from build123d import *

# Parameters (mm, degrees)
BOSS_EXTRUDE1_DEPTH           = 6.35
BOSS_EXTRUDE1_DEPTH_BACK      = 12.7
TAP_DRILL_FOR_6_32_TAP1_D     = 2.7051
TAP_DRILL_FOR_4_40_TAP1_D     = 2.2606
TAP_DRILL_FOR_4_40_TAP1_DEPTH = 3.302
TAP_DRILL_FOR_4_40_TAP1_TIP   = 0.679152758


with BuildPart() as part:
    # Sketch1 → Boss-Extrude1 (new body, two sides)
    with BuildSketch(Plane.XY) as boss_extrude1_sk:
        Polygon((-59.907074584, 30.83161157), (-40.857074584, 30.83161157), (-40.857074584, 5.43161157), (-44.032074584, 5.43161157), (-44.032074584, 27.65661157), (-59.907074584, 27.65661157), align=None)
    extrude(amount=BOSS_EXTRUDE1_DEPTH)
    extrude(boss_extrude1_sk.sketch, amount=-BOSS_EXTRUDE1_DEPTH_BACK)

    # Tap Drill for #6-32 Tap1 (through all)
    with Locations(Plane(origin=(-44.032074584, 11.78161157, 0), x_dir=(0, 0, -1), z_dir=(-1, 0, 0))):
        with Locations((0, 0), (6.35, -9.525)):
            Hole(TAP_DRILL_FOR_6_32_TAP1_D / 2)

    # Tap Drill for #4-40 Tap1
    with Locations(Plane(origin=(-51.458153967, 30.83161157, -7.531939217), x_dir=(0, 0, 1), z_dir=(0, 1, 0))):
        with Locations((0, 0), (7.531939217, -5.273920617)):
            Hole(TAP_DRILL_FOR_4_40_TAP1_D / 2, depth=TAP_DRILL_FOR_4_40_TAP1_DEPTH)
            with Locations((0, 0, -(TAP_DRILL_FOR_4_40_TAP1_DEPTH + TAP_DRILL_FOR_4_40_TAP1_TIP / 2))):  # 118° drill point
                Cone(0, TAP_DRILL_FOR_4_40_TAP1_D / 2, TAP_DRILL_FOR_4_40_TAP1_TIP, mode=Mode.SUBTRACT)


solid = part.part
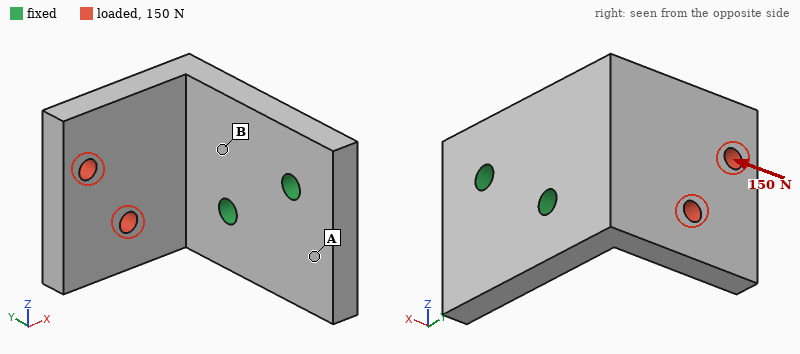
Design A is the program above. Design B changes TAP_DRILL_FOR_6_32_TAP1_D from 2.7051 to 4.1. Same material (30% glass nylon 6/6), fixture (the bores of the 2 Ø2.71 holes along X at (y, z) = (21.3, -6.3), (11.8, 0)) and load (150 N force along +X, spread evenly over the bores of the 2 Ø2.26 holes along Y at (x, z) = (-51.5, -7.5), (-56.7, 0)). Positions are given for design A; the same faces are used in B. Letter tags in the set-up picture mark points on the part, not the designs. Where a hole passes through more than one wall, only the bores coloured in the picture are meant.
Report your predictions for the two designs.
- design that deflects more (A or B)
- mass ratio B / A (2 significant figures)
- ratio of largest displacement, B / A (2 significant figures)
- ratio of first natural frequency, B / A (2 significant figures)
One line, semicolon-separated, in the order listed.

A; 0.98; 0.78; 1.1
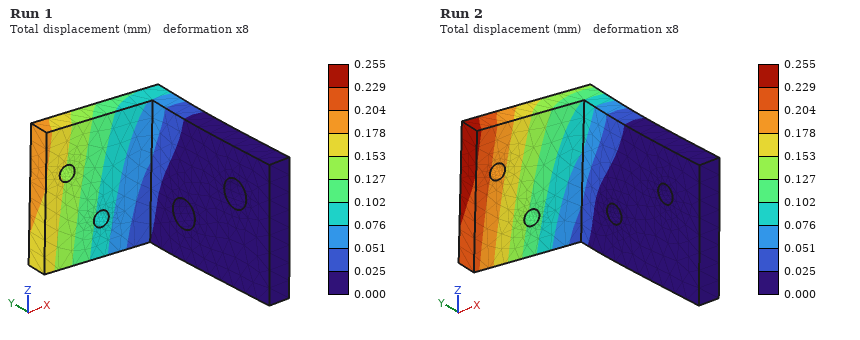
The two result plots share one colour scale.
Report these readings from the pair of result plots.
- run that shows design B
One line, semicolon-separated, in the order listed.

Run 1
